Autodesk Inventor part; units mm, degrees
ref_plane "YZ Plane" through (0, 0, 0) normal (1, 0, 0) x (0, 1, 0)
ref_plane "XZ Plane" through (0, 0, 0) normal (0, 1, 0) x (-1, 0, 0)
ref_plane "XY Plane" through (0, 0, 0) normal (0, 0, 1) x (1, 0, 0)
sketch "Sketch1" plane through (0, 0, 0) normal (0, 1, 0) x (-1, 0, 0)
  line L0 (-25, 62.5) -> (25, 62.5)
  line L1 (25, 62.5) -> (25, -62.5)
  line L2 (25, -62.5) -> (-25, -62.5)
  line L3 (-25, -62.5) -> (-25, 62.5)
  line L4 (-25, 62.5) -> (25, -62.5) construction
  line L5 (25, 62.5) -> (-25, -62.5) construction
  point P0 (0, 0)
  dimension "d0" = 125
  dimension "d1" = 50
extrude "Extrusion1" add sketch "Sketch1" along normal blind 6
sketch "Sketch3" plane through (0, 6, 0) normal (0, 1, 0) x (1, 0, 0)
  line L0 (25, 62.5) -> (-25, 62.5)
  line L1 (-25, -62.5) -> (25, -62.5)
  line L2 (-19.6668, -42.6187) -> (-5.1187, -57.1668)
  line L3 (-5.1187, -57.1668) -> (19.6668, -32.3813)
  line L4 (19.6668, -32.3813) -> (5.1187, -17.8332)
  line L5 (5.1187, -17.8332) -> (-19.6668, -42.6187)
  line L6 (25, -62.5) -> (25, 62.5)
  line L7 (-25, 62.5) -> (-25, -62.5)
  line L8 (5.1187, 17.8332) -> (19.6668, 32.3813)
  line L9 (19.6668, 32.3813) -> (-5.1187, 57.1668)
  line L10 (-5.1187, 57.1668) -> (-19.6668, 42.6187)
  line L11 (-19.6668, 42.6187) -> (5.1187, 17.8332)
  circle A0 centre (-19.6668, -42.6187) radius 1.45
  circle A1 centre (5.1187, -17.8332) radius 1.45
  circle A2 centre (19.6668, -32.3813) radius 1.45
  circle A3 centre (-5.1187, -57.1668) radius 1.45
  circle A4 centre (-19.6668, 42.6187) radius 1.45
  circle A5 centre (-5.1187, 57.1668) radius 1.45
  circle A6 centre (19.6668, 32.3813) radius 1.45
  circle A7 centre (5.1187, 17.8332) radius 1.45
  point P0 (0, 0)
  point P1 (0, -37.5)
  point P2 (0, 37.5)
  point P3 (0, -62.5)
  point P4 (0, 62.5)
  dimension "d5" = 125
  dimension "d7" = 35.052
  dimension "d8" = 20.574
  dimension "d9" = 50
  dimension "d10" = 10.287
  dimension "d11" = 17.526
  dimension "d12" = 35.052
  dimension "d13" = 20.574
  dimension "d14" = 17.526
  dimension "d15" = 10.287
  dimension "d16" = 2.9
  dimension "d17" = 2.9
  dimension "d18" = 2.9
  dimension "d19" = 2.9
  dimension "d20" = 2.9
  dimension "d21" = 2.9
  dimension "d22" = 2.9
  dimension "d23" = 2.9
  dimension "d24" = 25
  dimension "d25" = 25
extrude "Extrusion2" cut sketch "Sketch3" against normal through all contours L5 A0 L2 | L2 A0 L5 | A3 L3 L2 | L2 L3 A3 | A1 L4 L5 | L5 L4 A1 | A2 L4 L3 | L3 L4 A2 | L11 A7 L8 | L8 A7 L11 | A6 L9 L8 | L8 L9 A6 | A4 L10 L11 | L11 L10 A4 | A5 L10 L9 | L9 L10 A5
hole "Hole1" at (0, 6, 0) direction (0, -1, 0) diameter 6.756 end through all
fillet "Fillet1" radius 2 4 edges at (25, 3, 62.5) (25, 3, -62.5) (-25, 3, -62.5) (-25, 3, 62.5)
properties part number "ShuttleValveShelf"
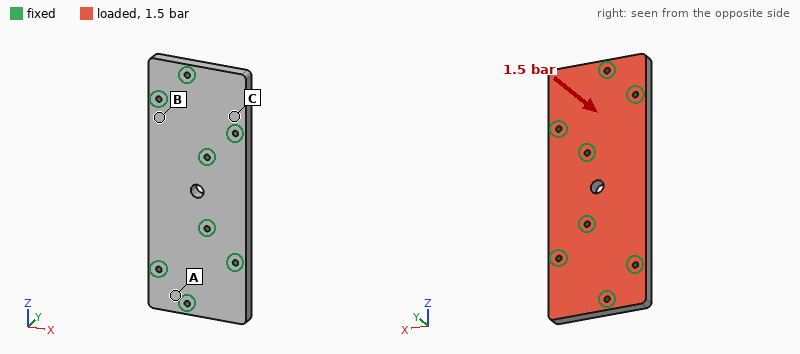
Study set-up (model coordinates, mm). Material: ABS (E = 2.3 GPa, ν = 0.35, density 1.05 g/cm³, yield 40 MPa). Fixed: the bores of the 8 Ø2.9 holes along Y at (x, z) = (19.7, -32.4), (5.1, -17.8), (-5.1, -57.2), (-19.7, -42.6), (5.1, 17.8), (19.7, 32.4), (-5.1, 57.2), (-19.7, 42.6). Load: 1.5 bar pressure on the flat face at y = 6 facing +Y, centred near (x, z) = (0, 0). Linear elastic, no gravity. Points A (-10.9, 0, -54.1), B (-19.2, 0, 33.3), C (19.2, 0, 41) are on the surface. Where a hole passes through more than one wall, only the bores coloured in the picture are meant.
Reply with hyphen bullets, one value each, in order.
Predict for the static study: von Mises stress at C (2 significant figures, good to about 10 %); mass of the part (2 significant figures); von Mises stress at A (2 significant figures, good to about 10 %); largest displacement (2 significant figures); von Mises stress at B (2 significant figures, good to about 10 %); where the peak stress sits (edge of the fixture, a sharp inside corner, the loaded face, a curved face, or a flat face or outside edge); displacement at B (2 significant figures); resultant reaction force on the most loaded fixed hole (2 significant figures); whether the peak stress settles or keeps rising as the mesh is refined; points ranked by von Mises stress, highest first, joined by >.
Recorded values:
- 1.9 MPa
- 39 g
- 1.0 MPa
- 0.26 mm
- 3.1 MPa
- edge of the fixture
- 0.047 mm
- 180 N
- keeps rising
- B > C > A
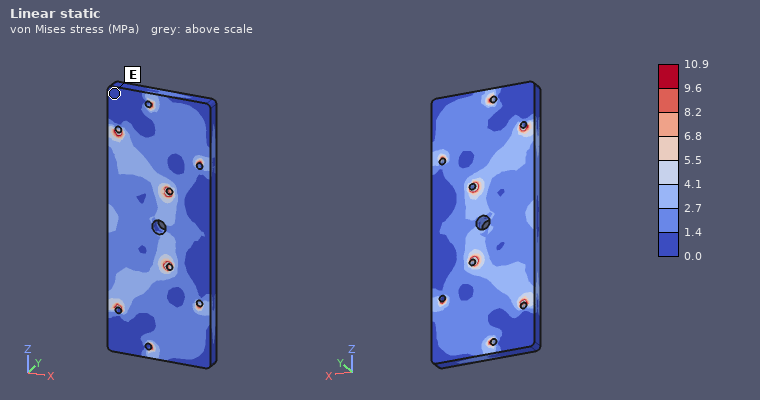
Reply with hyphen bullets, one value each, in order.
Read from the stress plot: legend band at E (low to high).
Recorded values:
- 0.0 to 1.4 MPa
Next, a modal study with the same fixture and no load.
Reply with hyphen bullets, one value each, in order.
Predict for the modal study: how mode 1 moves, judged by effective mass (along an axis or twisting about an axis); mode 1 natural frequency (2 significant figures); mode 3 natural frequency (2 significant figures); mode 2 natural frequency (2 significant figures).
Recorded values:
- along Y
- 2000 Hz
- 2800 Hz
- 2800 Hz
